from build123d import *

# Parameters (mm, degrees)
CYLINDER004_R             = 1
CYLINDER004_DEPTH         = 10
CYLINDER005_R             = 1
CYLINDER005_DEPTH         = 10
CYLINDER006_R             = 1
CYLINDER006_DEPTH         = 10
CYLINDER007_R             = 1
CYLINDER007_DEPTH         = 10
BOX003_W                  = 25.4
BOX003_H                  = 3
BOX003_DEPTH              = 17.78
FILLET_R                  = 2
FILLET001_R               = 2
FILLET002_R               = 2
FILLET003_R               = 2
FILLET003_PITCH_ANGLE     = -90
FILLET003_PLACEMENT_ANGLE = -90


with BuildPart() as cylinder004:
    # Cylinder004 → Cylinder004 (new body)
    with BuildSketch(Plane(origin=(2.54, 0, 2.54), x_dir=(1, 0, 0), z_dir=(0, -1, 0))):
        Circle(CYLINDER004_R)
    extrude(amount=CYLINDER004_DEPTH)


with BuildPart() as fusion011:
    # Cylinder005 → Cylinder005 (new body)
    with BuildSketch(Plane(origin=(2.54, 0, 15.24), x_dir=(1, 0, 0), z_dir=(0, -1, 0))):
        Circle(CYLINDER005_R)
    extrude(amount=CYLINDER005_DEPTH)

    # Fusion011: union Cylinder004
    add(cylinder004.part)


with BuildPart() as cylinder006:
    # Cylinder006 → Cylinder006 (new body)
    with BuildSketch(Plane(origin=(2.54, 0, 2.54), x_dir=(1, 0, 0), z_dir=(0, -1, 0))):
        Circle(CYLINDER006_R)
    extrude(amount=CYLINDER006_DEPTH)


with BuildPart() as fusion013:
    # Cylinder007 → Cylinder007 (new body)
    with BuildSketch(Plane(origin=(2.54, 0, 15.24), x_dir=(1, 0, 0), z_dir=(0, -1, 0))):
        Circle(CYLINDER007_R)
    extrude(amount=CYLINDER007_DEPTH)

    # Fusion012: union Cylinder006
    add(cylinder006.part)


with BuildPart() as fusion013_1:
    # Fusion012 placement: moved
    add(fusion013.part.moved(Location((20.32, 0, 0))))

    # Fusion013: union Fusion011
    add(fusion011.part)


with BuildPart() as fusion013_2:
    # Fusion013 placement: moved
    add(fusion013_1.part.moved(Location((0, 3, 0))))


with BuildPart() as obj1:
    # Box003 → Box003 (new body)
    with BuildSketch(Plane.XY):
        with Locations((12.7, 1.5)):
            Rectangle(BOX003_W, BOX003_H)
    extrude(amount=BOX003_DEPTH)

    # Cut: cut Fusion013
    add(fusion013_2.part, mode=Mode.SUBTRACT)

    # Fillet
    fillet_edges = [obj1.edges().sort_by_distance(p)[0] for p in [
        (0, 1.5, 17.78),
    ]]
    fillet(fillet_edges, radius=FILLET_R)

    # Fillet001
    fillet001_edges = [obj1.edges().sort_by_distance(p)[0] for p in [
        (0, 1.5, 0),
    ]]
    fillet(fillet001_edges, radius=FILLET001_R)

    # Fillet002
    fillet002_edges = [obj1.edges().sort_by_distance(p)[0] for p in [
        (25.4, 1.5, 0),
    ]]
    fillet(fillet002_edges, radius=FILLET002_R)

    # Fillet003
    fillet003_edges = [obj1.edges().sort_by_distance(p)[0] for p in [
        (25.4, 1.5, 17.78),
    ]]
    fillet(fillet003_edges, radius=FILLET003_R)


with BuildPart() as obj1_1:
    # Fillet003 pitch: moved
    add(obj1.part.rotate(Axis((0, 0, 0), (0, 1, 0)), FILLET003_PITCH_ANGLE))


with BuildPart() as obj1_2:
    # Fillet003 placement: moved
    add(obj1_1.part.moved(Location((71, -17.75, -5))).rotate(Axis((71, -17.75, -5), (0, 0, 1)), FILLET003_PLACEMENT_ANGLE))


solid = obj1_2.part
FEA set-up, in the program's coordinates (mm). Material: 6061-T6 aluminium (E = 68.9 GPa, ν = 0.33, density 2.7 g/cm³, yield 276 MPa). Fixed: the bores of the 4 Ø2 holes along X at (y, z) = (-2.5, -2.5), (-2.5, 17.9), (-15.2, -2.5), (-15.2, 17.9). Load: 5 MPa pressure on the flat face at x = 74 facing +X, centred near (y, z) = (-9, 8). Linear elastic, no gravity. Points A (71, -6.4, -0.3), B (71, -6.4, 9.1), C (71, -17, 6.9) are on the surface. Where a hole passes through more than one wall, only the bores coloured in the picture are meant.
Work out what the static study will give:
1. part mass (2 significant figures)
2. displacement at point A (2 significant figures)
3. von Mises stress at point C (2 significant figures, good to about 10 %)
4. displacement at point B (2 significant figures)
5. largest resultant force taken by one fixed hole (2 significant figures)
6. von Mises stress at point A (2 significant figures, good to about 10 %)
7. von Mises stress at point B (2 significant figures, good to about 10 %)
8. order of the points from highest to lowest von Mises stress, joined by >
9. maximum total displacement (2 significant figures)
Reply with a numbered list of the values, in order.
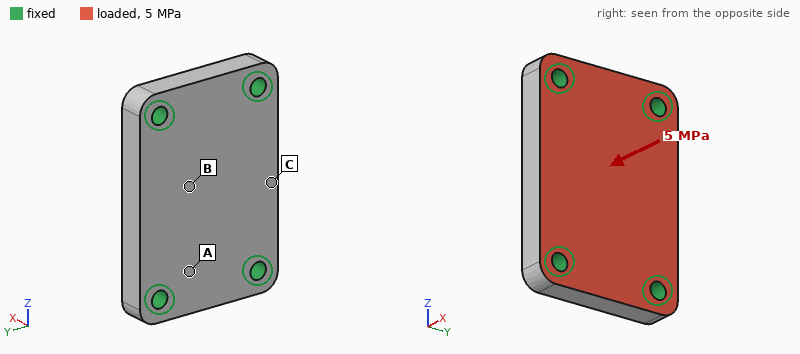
1. 3.5 g
2. 8.2 µm
3. 65 MPa
4. 20 µm
5. 550 N
6. 23 MPa
7. 52 MPa
8. C > B > A
9. 21 µm
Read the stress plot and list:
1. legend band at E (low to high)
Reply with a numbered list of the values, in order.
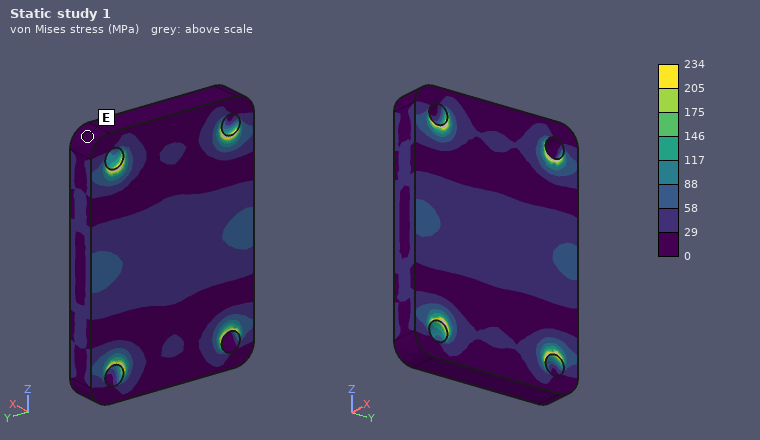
1. 0 to 29 MPa
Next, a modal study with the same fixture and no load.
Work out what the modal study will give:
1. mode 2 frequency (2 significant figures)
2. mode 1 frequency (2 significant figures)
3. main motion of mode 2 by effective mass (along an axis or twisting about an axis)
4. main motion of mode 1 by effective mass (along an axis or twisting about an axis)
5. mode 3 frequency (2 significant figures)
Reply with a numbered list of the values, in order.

1. 42 kHz
2. 31 kHz
3. twisting about Z
4. along X
5. 65 kHz
